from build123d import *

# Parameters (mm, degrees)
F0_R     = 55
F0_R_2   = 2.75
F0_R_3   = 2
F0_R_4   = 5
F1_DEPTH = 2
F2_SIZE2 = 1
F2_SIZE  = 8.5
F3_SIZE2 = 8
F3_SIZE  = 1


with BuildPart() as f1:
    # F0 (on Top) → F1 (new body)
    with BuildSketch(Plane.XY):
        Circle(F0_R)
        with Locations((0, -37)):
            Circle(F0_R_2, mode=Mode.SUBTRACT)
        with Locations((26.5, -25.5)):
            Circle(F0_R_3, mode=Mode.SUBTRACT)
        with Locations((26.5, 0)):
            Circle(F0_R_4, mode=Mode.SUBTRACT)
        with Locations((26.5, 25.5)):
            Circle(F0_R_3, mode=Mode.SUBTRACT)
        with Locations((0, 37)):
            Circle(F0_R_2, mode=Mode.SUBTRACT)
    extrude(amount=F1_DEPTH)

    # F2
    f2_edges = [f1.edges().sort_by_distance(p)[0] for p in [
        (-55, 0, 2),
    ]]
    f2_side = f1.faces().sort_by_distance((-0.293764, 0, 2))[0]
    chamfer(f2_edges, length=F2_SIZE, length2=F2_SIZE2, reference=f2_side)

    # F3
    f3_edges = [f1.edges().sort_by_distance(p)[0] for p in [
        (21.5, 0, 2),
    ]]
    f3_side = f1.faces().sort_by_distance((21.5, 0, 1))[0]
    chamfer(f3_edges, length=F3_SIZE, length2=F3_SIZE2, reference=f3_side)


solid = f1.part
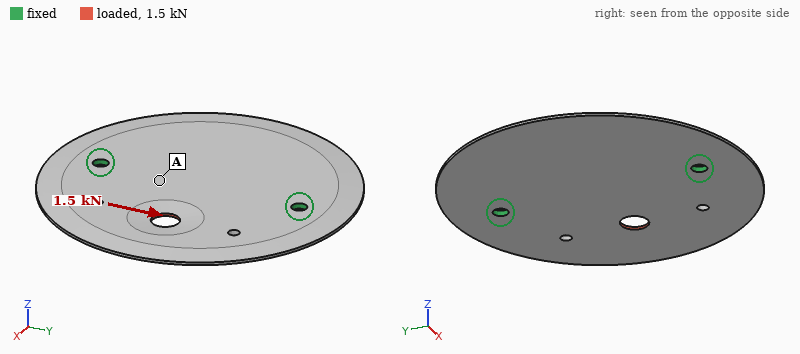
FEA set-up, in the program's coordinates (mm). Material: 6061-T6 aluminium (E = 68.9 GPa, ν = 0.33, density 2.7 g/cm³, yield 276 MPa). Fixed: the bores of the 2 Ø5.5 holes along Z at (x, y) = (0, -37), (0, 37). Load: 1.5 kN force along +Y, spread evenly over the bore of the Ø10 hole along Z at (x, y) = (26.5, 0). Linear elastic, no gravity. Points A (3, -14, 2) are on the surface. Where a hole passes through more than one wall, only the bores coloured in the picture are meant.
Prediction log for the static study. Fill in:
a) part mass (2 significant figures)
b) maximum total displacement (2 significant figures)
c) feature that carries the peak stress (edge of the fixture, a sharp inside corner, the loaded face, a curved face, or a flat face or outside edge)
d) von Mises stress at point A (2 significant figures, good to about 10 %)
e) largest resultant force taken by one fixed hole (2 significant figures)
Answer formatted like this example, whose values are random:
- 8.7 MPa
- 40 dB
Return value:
- 46 g
- 50 µm
- the loaded face
- 8.3 MPa
- 910 N
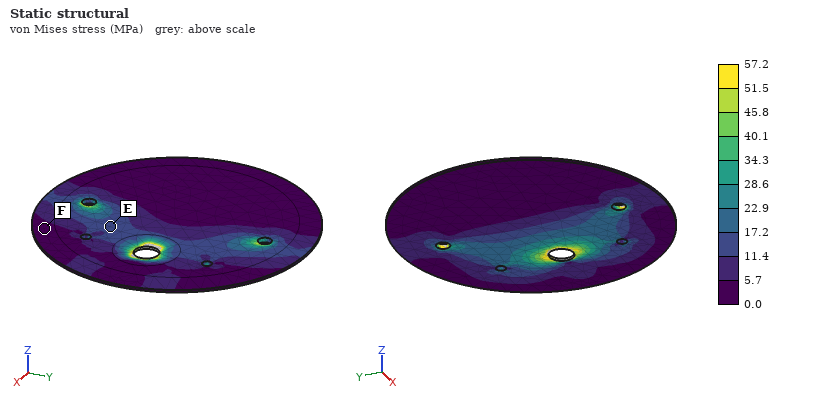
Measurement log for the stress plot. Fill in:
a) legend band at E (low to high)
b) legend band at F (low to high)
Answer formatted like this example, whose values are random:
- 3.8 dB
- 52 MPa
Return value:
- 11.4 to 17.2 MPa
- 0.0 to 5.7 MPa
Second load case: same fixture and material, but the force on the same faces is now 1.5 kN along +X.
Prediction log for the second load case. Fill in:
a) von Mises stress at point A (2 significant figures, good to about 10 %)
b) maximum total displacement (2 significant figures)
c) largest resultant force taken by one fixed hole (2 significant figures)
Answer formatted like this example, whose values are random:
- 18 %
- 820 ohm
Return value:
- 5.2 MPa
- 0.26 mm
- 770 N
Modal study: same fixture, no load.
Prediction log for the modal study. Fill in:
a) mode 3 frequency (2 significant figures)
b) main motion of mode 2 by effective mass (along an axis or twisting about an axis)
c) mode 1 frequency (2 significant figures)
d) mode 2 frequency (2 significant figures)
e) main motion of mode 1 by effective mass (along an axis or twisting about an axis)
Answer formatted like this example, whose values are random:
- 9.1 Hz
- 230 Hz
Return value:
- 1500 Hz
- along Z
- 570 Hz
- 720 Hz
- twisting about Y
